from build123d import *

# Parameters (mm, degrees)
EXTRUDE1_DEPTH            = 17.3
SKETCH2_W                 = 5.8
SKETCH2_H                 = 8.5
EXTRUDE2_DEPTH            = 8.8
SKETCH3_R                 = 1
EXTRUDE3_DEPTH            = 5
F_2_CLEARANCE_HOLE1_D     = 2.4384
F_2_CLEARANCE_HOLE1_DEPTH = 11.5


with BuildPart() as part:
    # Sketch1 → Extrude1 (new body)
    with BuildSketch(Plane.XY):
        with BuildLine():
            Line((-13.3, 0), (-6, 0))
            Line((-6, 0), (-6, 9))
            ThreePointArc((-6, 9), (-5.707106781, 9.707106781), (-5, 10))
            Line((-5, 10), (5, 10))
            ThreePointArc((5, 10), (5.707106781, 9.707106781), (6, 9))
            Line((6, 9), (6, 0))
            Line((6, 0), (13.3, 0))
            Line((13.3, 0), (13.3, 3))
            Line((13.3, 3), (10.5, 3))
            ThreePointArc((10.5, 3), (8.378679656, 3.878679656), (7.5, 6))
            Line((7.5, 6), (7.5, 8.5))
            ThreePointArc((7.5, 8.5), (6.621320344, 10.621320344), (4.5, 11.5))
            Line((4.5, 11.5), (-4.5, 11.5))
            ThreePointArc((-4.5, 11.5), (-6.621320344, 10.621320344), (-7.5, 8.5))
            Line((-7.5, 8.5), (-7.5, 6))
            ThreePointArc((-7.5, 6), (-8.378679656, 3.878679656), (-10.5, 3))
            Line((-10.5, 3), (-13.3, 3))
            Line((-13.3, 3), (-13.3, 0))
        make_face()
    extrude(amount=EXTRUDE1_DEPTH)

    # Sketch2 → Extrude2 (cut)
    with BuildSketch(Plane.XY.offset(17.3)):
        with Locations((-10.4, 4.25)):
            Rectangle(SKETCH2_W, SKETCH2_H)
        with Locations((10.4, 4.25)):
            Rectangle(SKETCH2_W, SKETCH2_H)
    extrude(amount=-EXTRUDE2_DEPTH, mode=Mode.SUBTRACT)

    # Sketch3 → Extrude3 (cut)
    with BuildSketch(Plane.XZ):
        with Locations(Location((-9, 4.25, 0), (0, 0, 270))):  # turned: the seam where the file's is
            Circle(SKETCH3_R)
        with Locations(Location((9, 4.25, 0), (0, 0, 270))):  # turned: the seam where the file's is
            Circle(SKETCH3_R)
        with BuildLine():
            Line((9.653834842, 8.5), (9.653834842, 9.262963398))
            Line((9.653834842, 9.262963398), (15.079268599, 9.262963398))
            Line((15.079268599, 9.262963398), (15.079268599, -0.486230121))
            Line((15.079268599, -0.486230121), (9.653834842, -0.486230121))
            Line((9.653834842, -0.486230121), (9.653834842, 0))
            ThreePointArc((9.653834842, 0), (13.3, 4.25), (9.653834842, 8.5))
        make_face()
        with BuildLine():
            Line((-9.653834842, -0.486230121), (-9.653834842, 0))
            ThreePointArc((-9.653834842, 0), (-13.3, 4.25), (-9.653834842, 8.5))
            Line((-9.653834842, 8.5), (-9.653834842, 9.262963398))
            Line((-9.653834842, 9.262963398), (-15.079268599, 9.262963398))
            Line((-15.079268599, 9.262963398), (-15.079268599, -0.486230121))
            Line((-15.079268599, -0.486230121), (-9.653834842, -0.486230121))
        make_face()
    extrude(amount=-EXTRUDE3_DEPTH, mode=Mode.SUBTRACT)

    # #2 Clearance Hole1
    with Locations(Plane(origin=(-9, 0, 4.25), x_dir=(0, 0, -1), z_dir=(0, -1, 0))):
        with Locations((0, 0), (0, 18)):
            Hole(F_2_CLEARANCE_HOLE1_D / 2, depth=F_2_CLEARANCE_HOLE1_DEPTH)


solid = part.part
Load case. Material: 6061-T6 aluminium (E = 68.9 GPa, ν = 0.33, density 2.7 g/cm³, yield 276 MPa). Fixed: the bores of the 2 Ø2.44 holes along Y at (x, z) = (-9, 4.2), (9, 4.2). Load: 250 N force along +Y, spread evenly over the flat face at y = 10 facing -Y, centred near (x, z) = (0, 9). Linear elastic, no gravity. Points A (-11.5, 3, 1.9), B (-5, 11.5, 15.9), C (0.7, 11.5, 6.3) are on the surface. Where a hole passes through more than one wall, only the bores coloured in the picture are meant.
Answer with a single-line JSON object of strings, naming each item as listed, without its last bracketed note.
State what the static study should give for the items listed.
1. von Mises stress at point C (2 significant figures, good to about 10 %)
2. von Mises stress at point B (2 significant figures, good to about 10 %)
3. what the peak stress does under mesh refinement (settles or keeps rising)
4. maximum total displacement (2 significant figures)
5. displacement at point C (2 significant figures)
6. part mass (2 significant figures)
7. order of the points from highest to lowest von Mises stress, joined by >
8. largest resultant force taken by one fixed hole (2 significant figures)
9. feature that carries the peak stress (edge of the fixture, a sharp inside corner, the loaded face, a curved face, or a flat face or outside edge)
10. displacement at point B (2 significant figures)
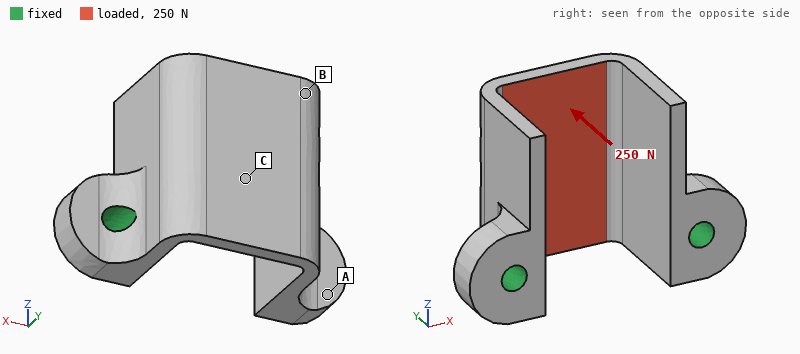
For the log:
{"von Mises stress at point C": "35 MPa", "von Mises stress at point B": "9.4 MPa", "what the peak stress does under mesh refinement": "keeps rising", "maximum total displacement": "23 µm", "displacement at point C": "12 µm", "part mass": "3.0 g", "order of the points from highest to lowest von Mises stress, joined by >": "C > B > A", "largest resultant force taken by one fixed hole": "140 N", "feature that carries the peak stress": "edge of the fixture", "displacement at point B": "12 µm"}
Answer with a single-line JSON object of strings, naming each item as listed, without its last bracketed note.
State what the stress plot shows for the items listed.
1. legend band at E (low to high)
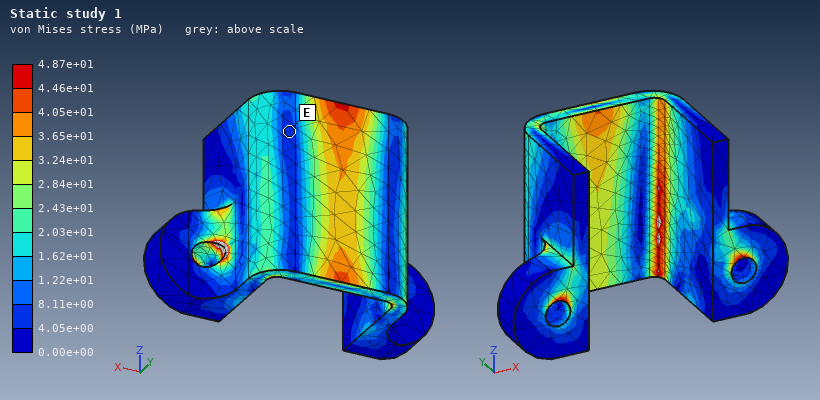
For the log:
{"legend band at E": "4.05e+00 to 8.11e+00 MPa"}
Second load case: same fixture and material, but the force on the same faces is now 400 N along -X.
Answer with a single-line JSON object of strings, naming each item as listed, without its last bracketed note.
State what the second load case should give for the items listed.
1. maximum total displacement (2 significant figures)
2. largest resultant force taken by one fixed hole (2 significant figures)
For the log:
{"maximum total displacement": "47 µm", "largest resultant force taken by one fixed hole": "230 N"}
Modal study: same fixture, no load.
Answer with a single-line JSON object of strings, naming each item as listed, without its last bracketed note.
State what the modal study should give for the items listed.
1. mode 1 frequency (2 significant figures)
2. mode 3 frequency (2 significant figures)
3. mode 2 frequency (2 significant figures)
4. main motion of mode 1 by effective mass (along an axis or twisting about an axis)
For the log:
{"mode 1 frequency": "13 kHz", "mode 3 frequency": "19 kHz", "mode 2 frequency": "16 kHz", "main motion of mode 1 by effective mass": "along X"}
